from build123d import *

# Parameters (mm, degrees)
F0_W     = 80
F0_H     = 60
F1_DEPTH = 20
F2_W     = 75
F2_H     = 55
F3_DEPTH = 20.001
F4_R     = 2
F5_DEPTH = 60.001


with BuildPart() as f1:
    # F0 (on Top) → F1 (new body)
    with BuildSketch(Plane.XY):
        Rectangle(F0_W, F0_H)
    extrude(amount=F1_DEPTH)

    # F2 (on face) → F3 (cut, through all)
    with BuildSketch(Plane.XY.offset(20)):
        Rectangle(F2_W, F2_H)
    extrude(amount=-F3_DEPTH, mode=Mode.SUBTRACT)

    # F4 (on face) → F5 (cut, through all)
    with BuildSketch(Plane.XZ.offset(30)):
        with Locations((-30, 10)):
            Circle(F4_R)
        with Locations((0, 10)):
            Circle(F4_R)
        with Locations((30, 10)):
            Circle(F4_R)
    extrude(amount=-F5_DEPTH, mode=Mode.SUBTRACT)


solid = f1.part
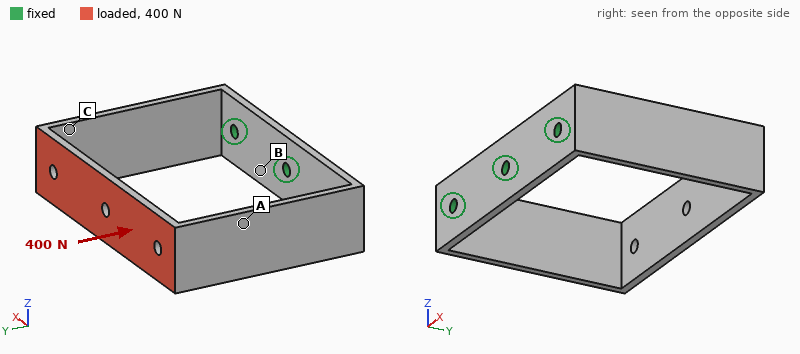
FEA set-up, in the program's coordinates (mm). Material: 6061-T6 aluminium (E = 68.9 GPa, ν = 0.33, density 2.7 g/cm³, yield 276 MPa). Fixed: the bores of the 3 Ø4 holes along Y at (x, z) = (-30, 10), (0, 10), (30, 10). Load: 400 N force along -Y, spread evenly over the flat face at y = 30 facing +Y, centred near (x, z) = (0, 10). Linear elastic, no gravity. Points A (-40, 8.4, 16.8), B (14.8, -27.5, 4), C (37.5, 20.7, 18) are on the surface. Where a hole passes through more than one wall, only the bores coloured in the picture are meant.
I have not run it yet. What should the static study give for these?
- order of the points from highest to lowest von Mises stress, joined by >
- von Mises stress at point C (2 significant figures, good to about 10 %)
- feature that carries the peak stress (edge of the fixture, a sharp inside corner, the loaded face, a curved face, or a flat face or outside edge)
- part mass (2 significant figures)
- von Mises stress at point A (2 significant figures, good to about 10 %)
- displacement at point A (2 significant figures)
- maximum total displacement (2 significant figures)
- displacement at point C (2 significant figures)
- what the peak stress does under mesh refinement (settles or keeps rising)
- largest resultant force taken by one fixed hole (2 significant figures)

C > A > B
75 MPa
edge of the fixture
36 g
45 MPa
0.17 mm
0.62 mm
0.12 mm
keeps rising
210 N
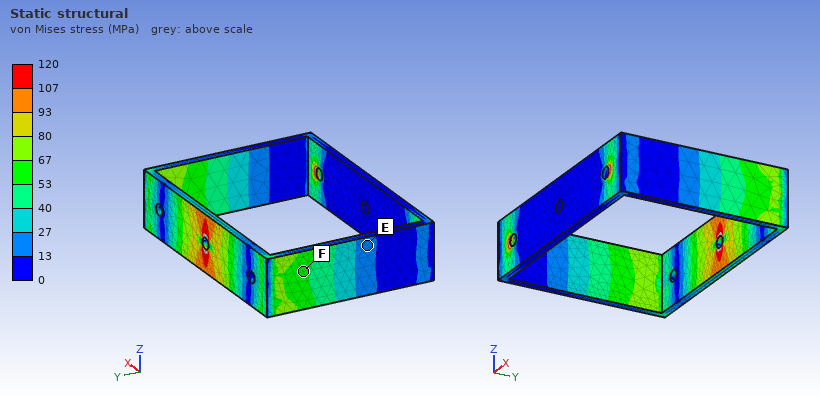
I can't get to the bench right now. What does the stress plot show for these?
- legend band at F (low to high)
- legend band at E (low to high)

53 to 67 MPa
13 to 27 MPa
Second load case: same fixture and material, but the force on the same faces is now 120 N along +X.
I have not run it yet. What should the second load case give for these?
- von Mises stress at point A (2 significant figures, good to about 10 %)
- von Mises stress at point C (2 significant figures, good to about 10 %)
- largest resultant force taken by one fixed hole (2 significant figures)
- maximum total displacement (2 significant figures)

18 MPa
53 MPa
78 N
1.1 mm
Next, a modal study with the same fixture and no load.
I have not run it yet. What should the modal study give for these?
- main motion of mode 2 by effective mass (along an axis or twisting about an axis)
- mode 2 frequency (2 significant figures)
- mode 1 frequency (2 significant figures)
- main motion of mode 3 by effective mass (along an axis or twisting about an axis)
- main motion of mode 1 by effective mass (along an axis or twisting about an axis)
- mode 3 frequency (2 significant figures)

along Z
630 Hz
420 Hz
twisting about Y
along X
1000 Hz
